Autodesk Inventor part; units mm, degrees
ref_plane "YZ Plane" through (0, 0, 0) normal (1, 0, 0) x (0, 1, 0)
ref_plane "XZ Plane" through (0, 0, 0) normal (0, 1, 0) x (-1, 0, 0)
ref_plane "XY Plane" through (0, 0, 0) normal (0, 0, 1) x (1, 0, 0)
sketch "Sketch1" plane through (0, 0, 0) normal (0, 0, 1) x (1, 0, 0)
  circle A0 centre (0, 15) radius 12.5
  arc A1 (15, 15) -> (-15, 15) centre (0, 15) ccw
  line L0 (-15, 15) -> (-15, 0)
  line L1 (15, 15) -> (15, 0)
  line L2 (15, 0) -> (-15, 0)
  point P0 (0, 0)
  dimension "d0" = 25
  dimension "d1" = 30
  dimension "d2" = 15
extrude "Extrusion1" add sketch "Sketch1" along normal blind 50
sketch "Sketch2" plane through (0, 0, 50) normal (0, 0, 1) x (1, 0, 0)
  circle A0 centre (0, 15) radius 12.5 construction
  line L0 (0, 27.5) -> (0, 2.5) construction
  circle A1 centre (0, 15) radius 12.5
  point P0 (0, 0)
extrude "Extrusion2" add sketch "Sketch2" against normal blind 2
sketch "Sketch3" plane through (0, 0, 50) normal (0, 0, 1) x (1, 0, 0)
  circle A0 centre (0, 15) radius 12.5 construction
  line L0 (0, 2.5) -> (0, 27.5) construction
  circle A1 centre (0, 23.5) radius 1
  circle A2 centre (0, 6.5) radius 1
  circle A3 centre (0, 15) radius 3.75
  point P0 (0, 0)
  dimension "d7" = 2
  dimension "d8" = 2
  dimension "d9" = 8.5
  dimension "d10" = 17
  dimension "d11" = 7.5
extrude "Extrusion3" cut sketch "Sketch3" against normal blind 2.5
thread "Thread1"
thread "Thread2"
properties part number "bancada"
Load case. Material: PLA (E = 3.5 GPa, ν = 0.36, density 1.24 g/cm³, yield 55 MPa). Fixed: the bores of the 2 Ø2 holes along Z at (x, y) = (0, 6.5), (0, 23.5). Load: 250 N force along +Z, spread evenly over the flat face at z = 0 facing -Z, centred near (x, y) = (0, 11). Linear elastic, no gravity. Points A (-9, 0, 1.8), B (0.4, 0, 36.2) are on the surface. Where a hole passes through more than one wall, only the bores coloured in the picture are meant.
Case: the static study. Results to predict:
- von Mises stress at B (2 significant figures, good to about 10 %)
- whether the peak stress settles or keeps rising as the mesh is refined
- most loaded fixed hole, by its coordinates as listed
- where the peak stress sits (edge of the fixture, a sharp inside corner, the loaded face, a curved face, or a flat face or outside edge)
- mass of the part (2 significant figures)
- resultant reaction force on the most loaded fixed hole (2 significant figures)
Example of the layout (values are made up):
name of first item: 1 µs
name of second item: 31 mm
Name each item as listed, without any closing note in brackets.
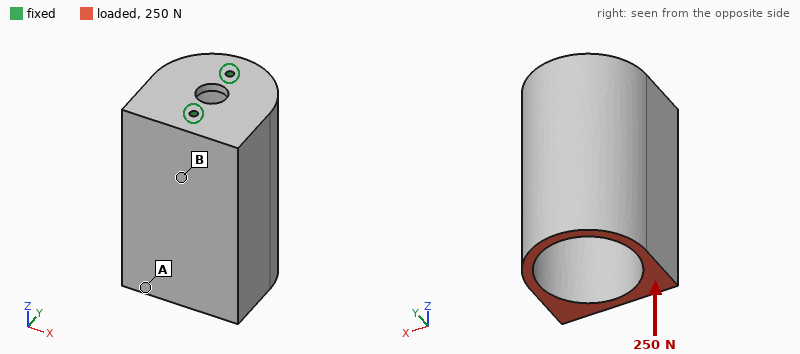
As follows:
von Mises stress at B: 2.8 MPa
whether the peak stress settles or keeps rising as the mesh is refined: keeps rising
most loaded fixed hole, by its coordinates as listed: (0, 6.5)
where the peak stress sits: edge of the fixture
mass of the part: 20 g
resultant reaction force on the most loaded fixed hole: 170 N
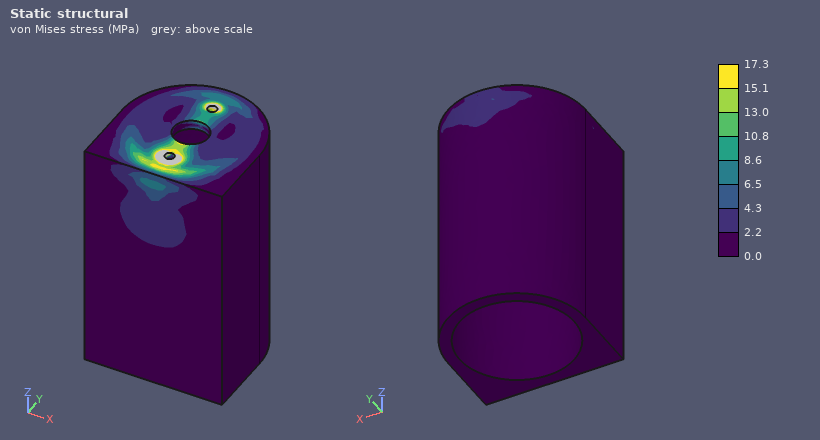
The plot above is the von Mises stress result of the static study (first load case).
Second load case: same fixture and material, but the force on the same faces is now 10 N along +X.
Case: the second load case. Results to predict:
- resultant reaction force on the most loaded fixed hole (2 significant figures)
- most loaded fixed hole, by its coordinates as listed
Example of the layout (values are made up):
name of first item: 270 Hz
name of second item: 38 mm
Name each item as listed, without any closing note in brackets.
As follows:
resultant reaction force on the most loaded fixed hole: 7.0 N
most loaded fixed hole, by its coordinates as listed: (0, 6.5)
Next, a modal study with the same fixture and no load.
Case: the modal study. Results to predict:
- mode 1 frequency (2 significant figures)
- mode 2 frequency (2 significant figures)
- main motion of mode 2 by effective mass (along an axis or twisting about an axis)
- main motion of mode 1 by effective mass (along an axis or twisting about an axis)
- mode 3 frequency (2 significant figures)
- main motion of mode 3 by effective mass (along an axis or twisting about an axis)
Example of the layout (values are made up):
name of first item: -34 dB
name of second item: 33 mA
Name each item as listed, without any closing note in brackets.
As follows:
mode 1 frequency: 220 Hz
mode 2 frequency: 670 Hz
main motion of mode 2 by effective mass: along Y
main motion of mode 1 by effective mass: along X
mode 3 frequency: 2000 Hz
main motion of mode 3 by effective mass: along Z
